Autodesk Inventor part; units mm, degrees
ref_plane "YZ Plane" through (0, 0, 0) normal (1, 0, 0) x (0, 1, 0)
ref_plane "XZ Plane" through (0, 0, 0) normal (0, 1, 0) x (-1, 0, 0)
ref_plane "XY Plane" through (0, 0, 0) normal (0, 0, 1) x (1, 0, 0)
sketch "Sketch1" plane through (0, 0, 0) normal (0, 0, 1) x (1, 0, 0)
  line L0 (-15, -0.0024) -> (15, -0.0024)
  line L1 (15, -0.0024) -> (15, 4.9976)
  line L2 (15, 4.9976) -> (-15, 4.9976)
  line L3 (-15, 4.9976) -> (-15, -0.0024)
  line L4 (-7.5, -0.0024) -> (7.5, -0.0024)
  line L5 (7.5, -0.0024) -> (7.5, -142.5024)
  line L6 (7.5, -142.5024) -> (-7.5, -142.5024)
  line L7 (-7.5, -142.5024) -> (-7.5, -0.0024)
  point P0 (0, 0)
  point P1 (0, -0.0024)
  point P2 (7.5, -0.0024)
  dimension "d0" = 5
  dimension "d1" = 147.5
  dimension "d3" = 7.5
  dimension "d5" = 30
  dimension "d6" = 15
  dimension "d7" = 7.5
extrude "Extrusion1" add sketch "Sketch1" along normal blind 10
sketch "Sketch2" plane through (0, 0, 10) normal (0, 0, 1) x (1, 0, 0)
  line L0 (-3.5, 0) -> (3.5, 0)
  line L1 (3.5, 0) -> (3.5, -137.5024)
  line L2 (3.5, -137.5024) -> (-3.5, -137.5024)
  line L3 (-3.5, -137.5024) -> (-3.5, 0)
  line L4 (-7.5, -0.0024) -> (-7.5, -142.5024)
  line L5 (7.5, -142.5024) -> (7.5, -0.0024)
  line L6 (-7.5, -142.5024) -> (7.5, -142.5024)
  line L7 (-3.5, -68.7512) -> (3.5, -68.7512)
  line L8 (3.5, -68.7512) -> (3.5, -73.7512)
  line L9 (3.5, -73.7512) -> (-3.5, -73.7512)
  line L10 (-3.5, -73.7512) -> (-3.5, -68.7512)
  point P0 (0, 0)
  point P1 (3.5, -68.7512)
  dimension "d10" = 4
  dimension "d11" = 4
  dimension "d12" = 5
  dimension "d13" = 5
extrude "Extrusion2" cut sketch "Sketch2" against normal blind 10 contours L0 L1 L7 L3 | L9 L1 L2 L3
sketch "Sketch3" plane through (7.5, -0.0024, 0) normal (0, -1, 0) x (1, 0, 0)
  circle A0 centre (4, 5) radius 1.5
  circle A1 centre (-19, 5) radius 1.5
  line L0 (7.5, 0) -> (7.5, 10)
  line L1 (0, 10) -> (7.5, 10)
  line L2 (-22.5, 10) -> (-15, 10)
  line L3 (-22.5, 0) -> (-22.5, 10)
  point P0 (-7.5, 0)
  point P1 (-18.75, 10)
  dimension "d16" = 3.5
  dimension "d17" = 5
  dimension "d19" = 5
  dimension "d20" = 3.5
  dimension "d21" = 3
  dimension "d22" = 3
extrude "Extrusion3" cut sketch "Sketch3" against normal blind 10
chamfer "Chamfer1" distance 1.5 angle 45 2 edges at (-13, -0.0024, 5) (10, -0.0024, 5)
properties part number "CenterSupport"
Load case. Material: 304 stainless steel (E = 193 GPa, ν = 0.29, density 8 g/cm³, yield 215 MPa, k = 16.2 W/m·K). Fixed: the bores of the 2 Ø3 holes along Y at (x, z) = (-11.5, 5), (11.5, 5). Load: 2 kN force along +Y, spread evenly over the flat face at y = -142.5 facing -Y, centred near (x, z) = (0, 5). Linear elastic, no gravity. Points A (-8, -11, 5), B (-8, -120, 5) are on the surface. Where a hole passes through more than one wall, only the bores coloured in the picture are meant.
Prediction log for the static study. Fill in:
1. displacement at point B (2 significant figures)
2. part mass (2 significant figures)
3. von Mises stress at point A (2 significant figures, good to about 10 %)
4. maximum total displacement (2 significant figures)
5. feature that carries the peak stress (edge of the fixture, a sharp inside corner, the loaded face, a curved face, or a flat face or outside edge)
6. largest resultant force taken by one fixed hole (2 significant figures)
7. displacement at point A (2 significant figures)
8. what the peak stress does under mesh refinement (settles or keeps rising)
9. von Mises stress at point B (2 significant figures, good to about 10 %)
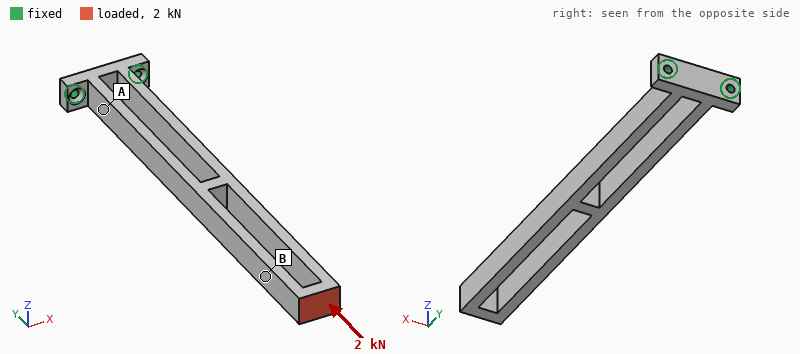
20 µm
110 g
34 MPa
24 µm
edge of the fixture
1.1 kN
7.3 µm
keeps rising
21 MPa
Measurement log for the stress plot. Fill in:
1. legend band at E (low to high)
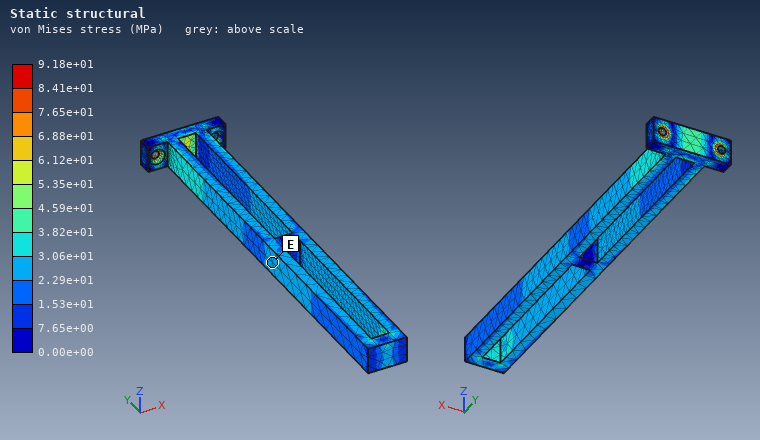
2.29e+01 to 3.06e+01 MPa
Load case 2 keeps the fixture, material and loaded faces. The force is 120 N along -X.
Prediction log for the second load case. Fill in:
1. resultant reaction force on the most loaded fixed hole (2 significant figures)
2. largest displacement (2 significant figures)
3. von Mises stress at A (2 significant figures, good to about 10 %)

900 N
0.60 mm
93 MPa
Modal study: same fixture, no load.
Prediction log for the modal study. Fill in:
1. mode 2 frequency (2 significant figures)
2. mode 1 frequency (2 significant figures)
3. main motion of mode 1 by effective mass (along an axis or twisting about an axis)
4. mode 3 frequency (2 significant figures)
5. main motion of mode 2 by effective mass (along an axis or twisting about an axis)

380 Hz
290 Hz
along Z
1300 Hz
along X
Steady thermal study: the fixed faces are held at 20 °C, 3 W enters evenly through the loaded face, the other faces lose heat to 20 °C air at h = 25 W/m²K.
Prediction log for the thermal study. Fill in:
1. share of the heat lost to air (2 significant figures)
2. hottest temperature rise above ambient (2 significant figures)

99 %
67 K
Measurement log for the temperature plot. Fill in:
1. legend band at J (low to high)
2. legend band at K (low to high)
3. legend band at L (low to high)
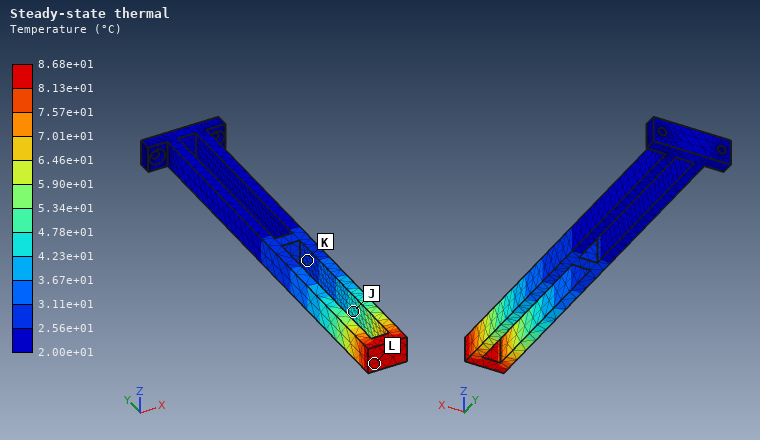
4.23e+01 to 4.78e+01 °C
2.56e+01 to 3.11e+01 °C
8.13e+01 to 8.68e+01 °C
